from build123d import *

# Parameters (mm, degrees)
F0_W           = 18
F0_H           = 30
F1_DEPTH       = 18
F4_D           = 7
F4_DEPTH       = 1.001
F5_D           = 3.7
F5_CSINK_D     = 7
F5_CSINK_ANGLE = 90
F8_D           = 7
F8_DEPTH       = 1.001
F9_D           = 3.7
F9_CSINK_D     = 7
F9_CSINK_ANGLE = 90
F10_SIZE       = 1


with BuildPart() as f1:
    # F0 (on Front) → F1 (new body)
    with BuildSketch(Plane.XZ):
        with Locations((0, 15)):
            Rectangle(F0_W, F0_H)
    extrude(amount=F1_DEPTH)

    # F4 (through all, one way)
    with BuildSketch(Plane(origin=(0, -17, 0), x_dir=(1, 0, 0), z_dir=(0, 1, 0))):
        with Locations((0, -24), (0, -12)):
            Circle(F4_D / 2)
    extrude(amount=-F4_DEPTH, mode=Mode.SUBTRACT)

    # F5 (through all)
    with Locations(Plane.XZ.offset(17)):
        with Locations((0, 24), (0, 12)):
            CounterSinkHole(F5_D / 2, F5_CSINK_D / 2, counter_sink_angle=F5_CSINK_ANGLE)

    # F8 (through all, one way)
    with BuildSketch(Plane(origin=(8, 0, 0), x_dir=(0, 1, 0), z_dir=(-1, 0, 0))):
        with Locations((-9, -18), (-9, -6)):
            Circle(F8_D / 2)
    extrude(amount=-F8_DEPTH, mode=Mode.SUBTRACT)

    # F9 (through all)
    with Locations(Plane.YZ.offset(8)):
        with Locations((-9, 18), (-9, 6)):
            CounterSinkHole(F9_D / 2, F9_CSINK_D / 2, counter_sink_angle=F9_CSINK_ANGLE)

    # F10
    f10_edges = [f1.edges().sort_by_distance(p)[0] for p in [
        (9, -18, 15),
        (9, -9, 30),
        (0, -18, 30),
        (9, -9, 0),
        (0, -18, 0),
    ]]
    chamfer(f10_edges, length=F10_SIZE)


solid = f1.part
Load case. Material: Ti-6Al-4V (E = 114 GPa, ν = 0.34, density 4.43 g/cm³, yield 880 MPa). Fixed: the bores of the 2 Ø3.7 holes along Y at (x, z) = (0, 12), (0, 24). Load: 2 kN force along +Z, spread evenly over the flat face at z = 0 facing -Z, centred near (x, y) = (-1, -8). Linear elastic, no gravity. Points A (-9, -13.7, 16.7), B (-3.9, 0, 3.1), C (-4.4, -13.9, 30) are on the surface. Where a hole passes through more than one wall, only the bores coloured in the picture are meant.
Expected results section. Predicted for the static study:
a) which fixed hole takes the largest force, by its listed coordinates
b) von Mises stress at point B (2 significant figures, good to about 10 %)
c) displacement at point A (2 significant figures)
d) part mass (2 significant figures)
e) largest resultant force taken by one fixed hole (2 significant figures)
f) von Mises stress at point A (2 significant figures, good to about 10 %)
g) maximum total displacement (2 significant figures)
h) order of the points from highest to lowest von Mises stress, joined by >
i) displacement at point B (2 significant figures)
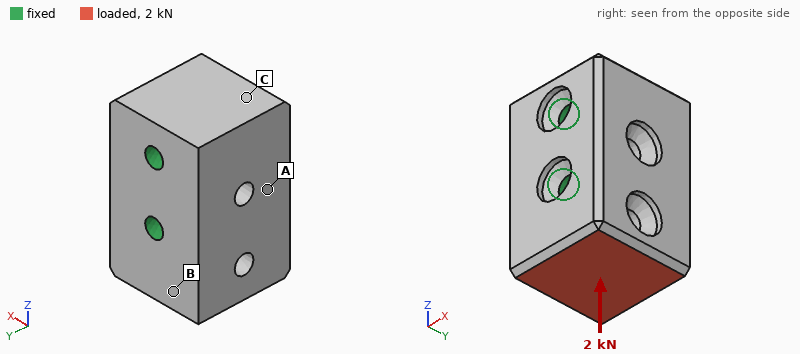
(0, 12)
6.9 MPa
0.33 µm
39 g
1.6 kN
3.9 MPa
1.4 µm
B > A > C
0.77 µm
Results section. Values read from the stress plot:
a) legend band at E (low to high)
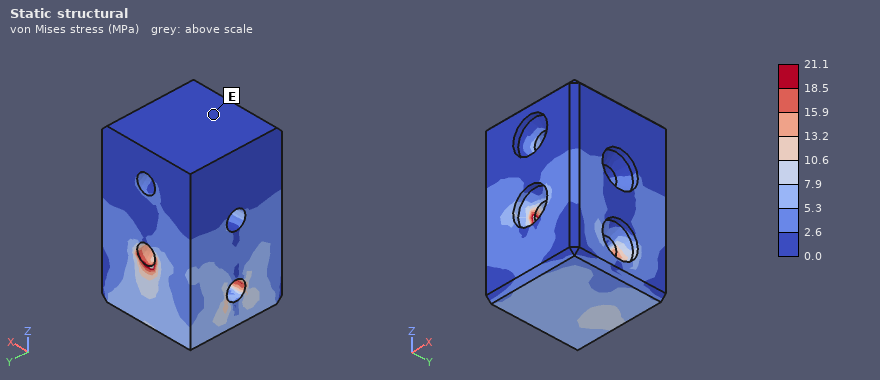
0.0 to 2.6 MPa
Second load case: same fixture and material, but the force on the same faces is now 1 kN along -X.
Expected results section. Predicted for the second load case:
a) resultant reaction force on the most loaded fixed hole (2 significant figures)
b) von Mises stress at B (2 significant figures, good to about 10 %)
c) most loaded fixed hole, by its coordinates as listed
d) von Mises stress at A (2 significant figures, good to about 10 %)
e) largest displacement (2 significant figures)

1.6 kN
8.9 MPa
(0, 12)
8.4 MPa
4.0 µm
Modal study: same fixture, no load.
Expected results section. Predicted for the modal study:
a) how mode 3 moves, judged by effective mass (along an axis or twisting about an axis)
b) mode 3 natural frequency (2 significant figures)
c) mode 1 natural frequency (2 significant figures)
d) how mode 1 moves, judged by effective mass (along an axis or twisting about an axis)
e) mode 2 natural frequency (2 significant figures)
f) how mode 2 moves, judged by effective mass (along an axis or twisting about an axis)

twisting about Z
46 kHz
34 kHz
along X
39 kHz
along Y
